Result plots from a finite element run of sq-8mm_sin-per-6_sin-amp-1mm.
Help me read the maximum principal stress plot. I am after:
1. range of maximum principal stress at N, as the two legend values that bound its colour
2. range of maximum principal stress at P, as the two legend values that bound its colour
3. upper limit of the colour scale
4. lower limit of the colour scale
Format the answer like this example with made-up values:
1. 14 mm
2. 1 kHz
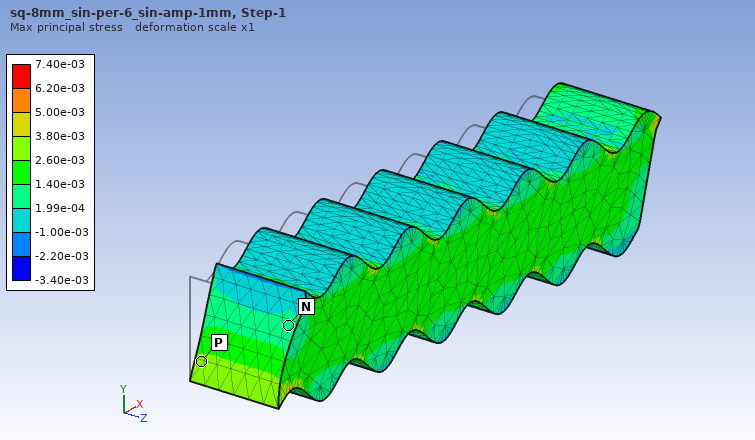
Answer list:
1. 1.99e-04 to 1.40e-03
2. 2.60e-03 to 3.80e-03
3. 7.40e-03
4. -3.40e-03
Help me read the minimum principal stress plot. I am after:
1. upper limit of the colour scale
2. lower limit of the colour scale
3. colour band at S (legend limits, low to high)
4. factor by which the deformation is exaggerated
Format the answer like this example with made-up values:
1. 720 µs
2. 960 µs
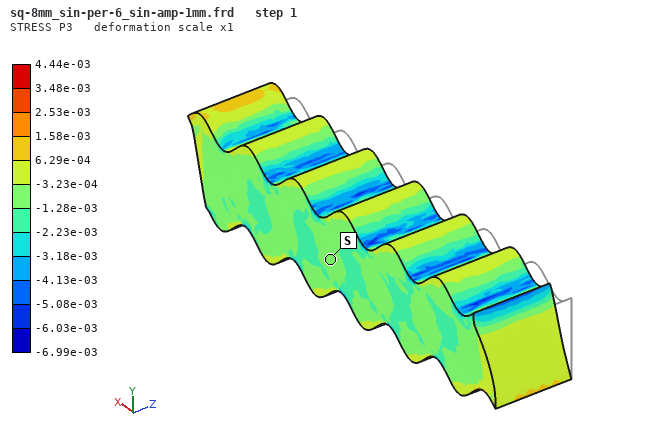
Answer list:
1. 4.44e-03
2. -6.99e-03
3. -1.28e-03 to -3.23e-04
4. 1
